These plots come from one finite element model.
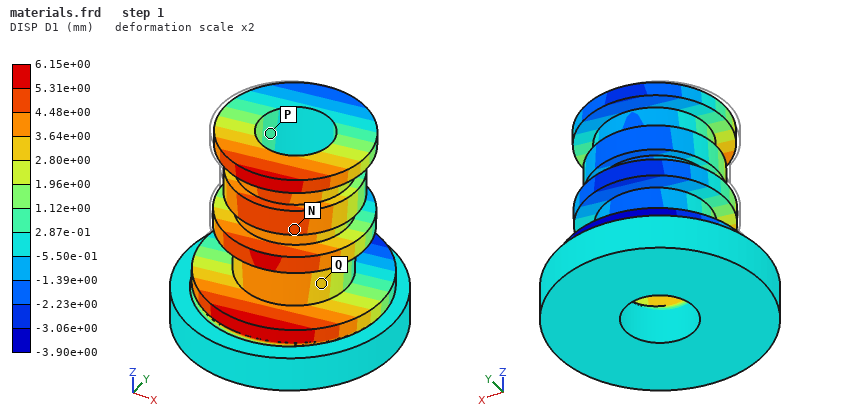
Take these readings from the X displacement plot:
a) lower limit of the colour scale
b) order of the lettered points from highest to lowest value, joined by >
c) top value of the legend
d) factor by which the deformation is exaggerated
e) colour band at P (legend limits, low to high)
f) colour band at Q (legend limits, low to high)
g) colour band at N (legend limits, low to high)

-3.90e+00 mm
N > Q > P
6.15e+00 mm
2
2.87e-01 to 1.12e+00 mm
2.80e+00 to 3.64e+00 mm
4.48e+00 to 5.31e+00 mm
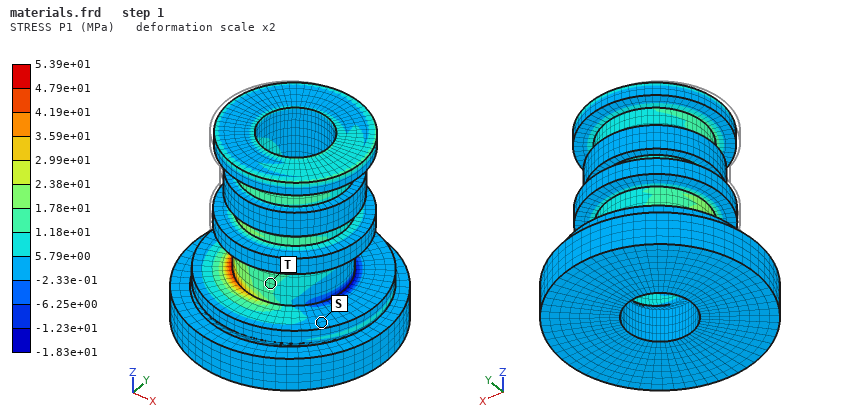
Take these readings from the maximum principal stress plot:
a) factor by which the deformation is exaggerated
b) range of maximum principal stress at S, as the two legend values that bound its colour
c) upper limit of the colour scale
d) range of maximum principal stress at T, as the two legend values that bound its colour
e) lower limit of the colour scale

2
-2.33e-01 to 5.79e+00 MPa
5.39e+01 MPa
1.18e+01 to 1.78e+01 MPa
-1.83e+01 MPa
